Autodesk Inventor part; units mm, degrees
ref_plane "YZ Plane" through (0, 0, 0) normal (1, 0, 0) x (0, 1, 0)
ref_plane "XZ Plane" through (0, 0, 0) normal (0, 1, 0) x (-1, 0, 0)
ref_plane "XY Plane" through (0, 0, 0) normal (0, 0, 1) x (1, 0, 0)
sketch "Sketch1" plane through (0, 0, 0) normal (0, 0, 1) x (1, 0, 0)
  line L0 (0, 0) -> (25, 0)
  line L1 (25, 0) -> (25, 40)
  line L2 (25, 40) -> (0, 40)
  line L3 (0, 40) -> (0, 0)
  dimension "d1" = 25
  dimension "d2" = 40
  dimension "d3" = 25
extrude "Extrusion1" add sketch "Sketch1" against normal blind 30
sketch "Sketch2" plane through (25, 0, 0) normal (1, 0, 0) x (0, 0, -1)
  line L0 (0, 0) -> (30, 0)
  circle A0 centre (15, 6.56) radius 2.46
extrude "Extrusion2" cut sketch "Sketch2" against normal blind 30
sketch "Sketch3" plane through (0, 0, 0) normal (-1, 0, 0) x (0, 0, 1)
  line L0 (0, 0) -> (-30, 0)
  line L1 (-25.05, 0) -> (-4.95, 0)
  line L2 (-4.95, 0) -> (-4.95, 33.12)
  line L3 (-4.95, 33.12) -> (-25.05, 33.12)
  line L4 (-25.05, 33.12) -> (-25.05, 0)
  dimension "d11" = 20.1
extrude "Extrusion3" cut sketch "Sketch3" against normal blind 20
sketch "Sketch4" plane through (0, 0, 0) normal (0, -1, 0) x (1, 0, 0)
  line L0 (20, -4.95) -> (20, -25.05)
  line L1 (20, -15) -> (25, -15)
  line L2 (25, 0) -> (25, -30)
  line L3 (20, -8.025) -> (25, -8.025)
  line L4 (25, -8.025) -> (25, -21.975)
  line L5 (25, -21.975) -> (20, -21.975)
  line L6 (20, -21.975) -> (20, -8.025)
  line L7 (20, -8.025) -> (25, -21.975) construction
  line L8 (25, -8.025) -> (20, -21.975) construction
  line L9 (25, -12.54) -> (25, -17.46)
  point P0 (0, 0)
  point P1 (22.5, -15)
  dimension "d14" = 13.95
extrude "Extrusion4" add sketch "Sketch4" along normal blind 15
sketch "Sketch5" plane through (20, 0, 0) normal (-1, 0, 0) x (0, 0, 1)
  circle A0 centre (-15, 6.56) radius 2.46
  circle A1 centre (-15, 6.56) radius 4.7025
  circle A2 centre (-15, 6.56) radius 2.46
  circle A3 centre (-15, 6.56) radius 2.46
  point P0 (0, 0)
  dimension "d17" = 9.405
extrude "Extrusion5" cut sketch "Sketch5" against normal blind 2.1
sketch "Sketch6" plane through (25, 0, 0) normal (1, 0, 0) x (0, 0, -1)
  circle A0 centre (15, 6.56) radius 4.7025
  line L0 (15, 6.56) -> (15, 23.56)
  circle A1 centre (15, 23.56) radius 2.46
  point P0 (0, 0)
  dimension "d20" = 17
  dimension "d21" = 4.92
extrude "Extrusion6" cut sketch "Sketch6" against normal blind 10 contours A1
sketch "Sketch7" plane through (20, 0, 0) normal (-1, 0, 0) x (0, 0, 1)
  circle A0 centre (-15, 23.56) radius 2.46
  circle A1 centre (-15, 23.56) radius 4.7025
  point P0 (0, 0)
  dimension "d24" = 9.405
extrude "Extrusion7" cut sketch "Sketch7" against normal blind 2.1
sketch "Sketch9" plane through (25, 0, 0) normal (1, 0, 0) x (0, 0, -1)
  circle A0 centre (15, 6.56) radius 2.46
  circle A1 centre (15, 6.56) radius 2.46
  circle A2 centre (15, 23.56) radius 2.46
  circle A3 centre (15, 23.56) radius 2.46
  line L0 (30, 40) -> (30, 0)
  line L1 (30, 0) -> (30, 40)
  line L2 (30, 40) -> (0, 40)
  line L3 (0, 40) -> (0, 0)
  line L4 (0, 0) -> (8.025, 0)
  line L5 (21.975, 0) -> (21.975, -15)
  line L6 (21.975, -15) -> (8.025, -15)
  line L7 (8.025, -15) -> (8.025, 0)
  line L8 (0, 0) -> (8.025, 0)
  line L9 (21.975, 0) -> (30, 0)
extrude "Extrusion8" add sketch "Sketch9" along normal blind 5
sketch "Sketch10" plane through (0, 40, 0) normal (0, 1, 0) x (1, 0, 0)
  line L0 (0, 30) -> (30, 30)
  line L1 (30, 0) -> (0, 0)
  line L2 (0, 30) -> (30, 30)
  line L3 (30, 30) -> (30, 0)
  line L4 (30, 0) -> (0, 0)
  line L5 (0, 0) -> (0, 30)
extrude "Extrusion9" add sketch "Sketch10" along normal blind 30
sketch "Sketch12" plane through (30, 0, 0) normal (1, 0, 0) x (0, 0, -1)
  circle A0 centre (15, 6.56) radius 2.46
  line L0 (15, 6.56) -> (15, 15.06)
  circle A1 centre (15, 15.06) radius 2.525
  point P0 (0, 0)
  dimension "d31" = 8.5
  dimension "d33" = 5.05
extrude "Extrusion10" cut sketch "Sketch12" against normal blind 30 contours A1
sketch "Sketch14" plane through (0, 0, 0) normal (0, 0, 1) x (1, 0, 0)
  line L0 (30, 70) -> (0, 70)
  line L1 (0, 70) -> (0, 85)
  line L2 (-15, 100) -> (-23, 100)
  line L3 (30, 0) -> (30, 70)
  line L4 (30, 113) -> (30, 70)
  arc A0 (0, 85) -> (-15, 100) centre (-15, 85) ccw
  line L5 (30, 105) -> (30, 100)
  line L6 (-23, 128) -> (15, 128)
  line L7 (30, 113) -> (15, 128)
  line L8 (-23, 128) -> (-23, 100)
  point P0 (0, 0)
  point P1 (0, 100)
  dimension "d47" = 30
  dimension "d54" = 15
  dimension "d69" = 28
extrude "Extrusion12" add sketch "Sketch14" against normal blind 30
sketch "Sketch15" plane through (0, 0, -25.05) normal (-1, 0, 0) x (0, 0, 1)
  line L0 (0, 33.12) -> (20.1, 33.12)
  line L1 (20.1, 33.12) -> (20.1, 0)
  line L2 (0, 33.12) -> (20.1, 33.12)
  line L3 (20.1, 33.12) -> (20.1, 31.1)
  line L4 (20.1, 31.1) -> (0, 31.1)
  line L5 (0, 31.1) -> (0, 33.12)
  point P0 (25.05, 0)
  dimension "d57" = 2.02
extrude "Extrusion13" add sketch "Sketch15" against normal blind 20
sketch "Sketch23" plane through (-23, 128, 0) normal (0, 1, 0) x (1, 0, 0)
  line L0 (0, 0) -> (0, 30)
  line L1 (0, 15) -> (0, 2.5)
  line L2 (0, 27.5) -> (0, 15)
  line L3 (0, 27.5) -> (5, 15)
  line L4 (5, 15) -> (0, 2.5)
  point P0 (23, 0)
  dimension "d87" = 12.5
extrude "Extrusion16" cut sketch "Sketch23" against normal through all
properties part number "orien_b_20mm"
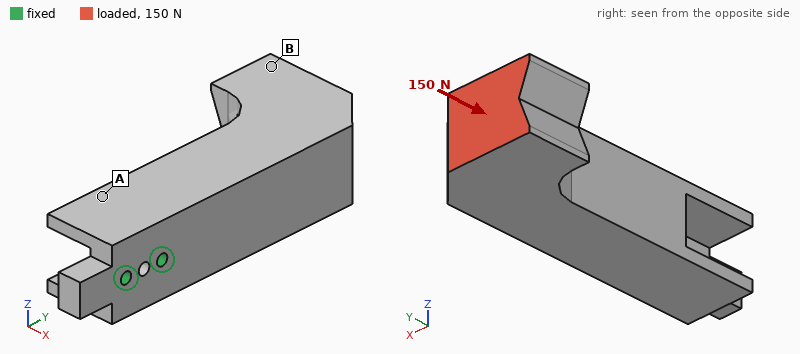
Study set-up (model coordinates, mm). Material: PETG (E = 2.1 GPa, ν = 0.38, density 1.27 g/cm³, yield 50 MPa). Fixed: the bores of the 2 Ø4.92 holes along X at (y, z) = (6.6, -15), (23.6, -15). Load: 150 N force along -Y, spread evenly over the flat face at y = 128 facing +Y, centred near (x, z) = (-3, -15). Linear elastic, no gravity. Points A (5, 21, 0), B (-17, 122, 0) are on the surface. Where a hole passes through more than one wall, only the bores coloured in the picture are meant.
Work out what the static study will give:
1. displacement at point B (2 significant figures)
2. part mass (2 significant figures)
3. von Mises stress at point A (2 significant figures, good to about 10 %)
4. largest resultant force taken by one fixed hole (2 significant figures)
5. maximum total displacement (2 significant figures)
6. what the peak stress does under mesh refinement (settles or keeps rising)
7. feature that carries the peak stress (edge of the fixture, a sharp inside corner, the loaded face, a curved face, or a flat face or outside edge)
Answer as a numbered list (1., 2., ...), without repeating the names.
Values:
1. 0.42 mm
2. 150 g
3. 1.1 MPa
4. 190 N
5. 0.46 mm
6. keeps rising
7. edge of the fixture
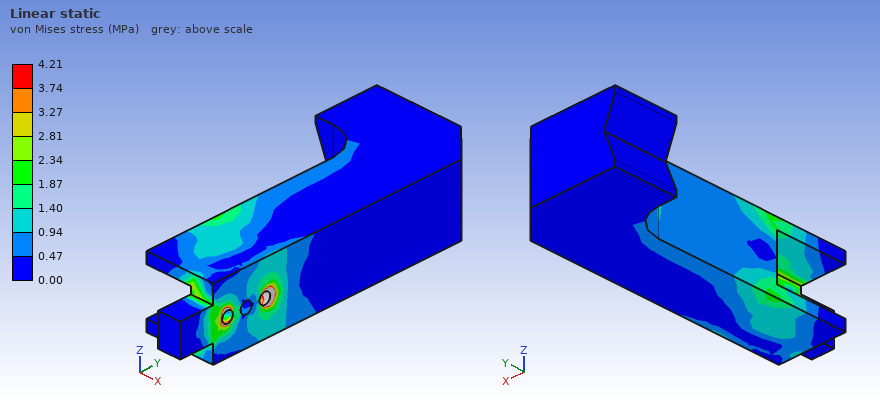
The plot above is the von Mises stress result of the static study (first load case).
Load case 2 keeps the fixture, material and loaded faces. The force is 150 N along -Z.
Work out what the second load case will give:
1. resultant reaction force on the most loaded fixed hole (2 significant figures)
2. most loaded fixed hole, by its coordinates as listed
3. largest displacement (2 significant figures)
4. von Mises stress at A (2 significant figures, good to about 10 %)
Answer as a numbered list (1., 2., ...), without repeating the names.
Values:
1. 830 N
2. (23.6, -15)
3. 1.4 mm
4. 2.3 MPa
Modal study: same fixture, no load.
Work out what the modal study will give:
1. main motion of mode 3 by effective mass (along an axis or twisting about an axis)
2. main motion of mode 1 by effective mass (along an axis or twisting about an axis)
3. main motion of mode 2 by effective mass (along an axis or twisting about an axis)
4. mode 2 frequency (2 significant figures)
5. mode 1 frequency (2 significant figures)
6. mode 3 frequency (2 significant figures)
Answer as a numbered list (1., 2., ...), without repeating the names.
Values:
1. twisting about Y
2. along X
3. along Z
4. 250 Hz
5. 210 Hz
6. 670 Hz
